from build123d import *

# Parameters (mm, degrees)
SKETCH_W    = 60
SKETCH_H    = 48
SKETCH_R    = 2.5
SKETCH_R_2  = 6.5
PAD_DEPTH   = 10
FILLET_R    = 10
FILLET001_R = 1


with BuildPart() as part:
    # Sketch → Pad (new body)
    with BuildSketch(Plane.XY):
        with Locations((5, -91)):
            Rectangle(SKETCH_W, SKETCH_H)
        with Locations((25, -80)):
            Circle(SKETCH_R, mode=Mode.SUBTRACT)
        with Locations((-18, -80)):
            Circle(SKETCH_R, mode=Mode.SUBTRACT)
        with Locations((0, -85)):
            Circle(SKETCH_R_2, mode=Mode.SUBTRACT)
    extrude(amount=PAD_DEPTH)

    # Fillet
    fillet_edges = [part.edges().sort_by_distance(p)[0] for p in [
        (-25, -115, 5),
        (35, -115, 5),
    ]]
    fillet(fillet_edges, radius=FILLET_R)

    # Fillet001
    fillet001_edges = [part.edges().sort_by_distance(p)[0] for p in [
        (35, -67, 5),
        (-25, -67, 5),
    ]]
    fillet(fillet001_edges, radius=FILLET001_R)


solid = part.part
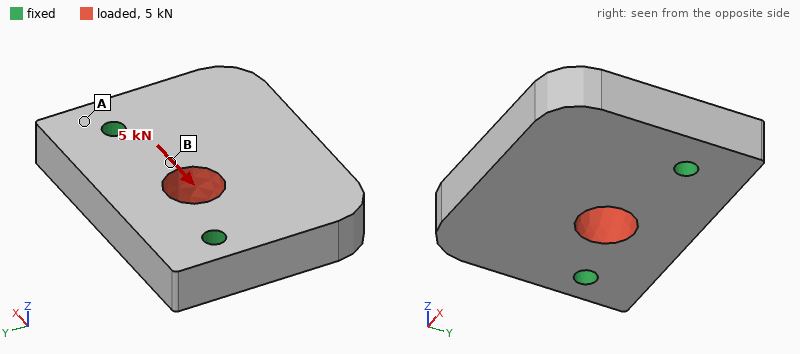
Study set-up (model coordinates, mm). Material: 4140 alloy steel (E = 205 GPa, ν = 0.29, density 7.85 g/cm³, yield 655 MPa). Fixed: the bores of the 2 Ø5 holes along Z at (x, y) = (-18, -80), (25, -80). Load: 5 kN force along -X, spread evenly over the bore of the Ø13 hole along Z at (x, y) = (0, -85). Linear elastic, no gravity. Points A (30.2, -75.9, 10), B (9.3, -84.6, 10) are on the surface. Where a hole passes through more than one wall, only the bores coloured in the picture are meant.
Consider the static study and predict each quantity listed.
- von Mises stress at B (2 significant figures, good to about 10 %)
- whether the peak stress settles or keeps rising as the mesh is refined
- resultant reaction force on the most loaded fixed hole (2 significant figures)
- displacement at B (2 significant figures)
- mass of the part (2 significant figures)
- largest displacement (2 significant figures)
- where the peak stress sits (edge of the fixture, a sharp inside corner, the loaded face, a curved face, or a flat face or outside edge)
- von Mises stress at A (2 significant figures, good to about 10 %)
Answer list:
14 MPa
keeps rising
2.7 kN
1.2 µm
210 g
1.9 µm
edge of the fixture
5.9 MPa
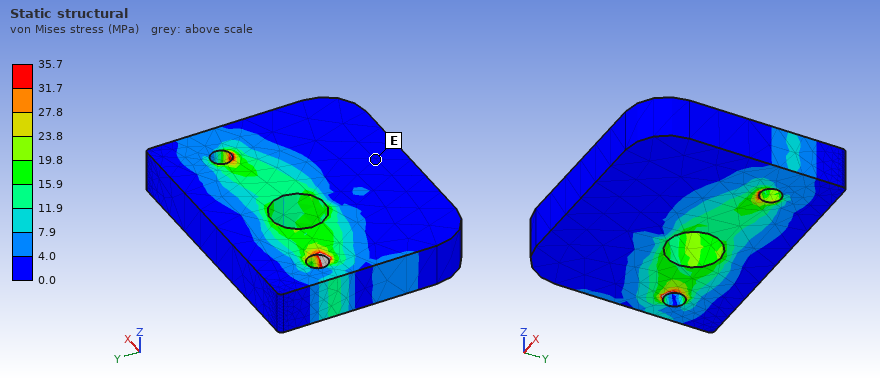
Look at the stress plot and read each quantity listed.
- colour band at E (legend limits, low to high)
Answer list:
0.0 to 4.0 MPa
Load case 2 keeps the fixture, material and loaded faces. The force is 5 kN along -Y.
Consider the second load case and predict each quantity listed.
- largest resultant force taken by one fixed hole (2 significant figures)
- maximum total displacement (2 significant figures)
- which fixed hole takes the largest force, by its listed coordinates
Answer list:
2.9 kN
2.7 µm
(-18, -80)
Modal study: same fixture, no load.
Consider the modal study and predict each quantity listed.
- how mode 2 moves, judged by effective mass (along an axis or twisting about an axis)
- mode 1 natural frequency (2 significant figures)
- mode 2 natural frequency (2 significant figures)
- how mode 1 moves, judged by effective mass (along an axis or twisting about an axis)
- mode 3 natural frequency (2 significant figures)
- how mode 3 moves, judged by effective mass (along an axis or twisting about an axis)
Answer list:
twisting about Y
5400 Hz
10 kHz
along Z
16 kHz
along X
